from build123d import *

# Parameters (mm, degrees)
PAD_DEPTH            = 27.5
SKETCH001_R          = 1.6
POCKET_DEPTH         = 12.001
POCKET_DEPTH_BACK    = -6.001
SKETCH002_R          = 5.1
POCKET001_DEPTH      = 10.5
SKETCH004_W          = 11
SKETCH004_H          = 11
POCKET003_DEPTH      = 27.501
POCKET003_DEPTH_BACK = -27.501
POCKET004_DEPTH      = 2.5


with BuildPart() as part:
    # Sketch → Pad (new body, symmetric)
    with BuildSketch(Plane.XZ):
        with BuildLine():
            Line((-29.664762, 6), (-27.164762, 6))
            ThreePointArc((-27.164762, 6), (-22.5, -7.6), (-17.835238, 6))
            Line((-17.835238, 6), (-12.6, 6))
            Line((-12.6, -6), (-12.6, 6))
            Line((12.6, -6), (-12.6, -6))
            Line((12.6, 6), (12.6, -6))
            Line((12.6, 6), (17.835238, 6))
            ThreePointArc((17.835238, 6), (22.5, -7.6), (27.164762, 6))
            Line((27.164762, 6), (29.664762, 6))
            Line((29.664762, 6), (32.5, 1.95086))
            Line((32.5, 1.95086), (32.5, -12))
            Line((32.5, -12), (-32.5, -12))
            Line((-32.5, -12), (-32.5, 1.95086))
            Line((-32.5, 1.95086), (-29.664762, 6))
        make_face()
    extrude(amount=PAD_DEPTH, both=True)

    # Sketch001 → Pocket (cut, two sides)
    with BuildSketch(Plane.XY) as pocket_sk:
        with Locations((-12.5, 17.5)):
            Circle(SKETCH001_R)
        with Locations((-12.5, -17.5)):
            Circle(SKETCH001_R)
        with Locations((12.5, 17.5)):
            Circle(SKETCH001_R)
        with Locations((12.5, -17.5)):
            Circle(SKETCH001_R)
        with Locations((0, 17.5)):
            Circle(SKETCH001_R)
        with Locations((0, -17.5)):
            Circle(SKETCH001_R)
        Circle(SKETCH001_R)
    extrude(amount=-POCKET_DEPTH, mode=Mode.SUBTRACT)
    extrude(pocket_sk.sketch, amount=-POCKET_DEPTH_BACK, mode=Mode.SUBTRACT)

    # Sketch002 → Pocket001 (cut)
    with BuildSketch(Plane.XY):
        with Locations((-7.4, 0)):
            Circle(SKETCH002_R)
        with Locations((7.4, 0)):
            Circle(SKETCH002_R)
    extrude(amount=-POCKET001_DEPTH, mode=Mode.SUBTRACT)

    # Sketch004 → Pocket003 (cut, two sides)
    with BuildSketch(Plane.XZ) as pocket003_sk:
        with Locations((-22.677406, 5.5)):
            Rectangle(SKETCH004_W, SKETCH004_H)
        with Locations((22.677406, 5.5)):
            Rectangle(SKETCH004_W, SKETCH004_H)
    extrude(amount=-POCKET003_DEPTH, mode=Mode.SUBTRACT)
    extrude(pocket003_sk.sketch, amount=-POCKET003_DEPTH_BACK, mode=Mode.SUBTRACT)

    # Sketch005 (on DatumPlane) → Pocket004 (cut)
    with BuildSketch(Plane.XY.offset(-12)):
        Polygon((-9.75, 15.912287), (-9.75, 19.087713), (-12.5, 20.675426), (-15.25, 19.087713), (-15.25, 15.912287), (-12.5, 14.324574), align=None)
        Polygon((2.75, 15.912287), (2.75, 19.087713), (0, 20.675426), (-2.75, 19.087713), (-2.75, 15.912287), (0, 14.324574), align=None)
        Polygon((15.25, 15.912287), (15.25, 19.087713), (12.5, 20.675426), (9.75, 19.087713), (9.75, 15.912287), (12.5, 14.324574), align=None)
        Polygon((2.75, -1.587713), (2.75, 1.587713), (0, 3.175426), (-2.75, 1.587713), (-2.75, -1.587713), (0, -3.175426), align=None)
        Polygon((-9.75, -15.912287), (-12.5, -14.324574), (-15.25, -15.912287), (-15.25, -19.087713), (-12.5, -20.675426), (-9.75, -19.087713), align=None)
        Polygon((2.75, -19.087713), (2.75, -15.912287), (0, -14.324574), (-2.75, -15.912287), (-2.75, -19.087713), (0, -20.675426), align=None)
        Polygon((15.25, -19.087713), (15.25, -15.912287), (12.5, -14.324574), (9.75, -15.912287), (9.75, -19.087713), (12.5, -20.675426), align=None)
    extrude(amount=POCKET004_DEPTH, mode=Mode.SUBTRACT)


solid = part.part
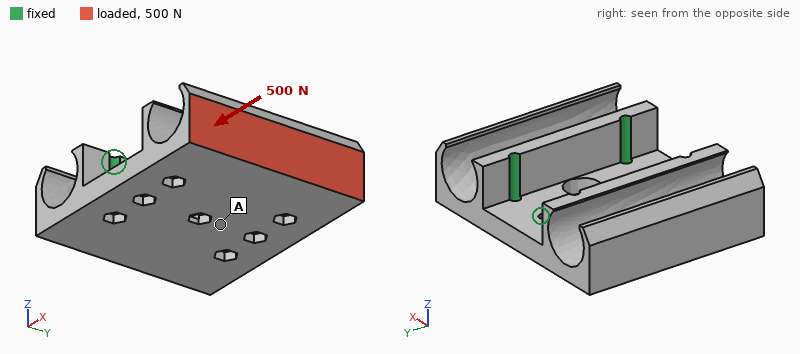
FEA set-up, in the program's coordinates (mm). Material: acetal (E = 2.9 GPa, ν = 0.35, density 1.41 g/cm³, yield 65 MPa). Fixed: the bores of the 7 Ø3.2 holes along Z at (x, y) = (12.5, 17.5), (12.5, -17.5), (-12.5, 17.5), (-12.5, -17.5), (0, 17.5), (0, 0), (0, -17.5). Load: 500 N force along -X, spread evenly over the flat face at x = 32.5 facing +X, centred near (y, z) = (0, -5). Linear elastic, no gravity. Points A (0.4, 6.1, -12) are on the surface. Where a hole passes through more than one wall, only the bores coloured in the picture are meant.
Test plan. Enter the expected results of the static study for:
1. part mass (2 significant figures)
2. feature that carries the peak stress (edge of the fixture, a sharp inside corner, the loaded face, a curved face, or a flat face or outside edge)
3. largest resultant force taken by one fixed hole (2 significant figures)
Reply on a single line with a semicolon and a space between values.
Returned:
38 g; a curved face; 200 N
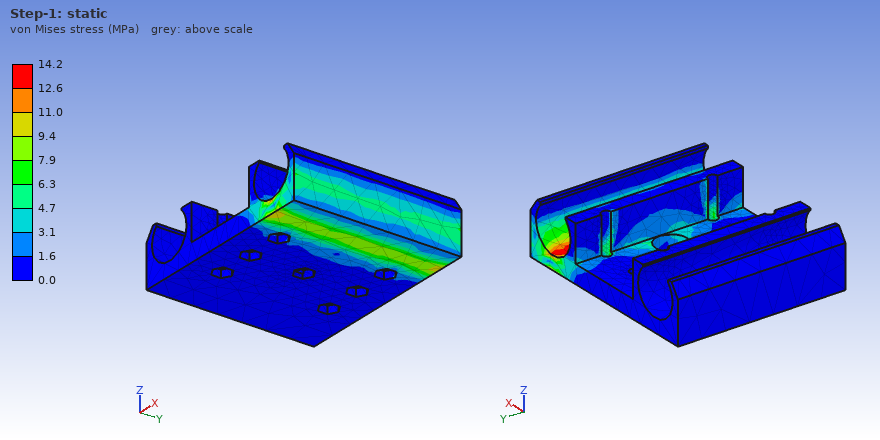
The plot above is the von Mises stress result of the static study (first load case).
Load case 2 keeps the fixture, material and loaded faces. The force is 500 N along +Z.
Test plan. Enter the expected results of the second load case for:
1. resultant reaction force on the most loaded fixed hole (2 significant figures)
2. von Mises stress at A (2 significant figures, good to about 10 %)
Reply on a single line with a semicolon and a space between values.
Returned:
470 N; 2.8 MPa
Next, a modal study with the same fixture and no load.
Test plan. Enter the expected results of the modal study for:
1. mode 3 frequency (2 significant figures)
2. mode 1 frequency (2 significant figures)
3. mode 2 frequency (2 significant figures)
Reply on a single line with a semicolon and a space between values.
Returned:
2600 Hz; 1900 Hz; 1900 Hz
